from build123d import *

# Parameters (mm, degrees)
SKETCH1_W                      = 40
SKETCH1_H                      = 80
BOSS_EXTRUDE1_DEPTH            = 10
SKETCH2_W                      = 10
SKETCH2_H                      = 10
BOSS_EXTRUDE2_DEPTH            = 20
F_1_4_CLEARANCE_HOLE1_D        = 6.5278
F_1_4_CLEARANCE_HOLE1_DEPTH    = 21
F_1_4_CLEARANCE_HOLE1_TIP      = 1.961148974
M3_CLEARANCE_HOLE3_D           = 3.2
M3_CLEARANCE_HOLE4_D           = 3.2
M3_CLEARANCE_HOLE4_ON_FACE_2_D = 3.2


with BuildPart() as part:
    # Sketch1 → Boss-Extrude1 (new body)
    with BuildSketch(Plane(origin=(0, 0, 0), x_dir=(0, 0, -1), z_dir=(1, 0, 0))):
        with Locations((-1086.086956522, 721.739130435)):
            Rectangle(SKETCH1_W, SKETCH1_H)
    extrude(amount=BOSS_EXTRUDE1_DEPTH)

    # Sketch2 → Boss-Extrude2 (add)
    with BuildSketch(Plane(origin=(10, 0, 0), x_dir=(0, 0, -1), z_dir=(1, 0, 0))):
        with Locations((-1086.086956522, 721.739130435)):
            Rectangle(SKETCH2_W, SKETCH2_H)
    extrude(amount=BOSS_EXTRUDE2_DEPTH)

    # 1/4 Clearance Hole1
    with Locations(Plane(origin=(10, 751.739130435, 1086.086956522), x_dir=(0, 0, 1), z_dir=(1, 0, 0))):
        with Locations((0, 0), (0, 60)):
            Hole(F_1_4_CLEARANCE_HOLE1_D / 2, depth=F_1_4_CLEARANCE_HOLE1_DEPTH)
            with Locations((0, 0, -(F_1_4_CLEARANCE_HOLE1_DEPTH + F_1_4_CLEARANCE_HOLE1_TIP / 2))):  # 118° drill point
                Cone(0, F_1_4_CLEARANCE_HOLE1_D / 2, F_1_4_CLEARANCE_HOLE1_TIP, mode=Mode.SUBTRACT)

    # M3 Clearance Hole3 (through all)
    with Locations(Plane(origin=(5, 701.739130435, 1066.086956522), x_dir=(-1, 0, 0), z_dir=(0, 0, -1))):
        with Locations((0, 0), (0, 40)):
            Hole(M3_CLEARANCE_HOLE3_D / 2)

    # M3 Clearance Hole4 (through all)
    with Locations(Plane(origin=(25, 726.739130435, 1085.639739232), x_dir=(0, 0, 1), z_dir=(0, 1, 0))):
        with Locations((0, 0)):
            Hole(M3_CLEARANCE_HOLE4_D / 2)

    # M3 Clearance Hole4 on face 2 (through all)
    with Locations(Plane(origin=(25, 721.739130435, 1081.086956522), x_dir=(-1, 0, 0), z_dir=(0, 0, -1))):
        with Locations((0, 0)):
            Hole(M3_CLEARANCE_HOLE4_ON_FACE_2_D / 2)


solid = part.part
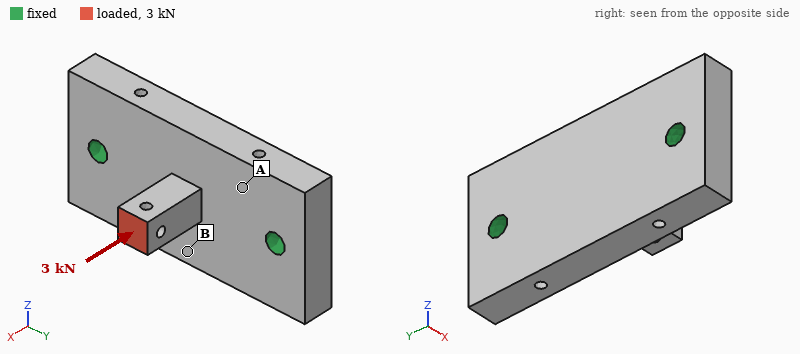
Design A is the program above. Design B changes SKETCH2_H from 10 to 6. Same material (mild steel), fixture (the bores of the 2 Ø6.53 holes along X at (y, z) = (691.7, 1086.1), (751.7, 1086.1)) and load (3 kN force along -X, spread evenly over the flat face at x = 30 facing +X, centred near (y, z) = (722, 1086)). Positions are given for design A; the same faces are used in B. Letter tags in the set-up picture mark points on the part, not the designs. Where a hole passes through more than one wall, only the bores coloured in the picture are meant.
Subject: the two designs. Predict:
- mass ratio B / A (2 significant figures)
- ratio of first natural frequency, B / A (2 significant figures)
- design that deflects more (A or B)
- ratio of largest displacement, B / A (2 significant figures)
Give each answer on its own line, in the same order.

0.98
1.1
B
1.4
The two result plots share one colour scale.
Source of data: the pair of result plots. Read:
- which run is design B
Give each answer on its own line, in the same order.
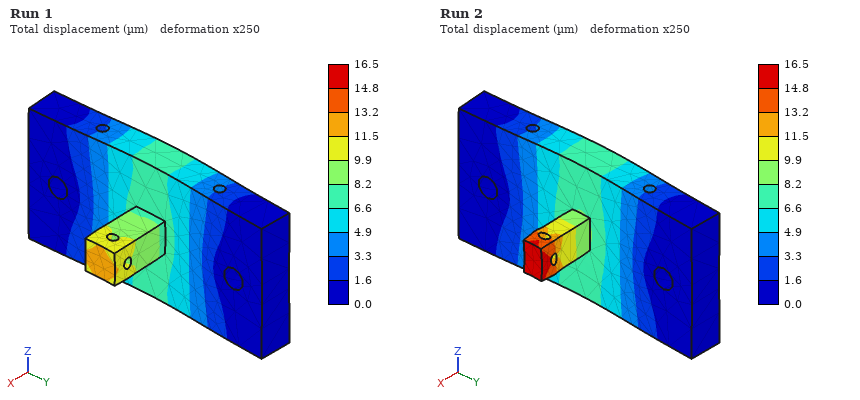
Run 2
